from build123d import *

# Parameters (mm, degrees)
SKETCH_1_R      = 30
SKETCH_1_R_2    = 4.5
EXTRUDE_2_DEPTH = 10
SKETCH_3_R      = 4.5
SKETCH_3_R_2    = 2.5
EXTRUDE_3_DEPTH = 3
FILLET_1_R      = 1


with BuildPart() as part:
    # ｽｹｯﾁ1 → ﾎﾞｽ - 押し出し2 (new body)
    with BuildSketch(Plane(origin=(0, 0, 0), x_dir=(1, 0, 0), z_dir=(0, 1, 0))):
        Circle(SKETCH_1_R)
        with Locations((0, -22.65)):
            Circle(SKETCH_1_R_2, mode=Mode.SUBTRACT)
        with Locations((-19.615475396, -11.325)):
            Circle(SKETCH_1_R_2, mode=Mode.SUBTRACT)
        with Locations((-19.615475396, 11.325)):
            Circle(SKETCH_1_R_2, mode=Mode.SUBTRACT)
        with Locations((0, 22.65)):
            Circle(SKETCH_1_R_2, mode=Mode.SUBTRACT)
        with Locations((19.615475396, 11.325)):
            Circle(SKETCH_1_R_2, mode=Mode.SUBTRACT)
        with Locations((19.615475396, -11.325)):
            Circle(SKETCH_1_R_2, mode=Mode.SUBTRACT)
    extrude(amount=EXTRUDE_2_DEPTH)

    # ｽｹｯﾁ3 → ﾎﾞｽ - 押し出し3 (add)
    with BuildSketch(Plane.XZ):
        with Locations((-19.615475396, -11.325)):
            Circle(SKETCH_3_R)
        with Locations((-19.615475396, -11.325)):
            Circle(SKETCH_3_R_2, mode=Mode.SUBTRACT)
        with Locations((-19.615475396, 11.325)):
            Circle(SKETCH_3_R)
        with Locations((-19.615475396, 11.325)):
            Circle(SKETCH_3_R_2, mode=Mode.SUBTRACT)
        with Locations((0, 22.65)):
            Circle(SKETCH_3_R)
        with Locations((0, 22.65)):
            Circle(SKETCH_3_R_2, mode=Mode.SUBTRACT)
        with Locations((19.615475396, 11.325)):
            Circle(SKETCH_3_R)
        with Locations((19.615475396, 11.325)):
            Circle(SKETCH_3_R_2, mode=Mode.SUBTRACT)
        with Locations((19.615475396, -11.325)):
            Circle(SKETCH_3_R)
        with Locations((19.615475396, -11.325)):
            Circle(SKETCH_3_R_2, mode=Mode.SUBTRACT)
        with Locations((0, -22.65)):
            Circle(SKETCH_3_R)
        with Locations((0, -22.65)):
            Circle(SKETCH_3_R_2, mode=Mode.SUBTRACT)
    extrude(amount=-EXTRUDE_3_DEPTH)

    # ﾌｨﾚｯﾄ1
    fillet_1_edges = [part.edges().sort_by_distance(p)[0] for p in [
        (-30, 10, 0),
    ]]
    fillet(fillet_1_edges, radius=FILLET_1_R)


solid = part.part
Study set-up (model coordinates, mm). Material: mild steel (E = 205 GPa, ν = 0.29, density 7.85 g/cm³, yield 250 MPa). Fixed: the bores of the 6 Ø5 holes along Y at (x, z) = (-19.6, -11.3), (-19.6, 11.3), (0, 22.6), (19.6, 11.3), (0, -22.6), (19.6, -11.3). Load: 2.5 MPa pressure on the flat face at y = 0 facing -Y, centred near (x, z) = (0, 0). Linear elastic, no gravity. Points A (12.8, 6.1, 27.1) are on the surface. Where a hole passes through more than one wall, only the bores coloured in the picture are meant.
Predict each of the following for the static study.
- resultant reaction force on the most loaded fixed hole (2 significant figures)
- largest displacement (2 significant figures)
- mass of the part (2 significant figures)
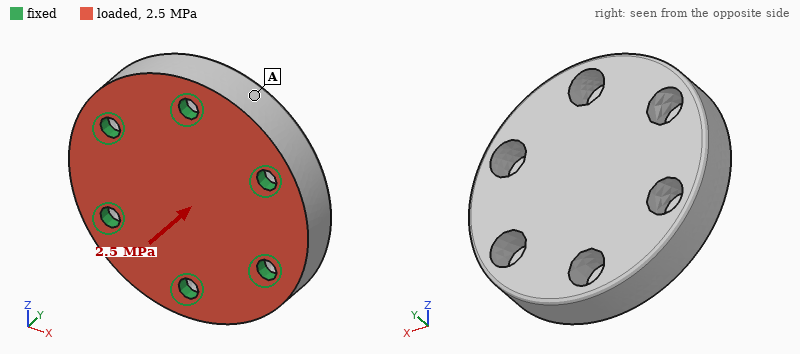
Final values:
1.1 kN
2.1 µm
200 g
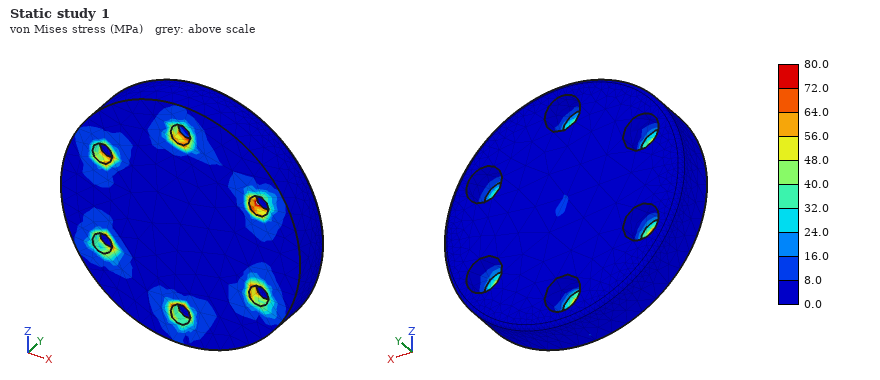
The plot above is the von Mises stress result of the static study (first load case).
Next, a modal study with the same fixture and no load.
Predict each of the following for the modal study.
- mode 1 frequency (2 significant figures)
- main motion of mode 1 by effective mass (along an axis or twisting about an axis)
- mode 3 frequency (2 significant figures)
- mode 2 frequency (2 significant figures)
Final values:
23 kHz
along Y
27 kHz
27 kHz
